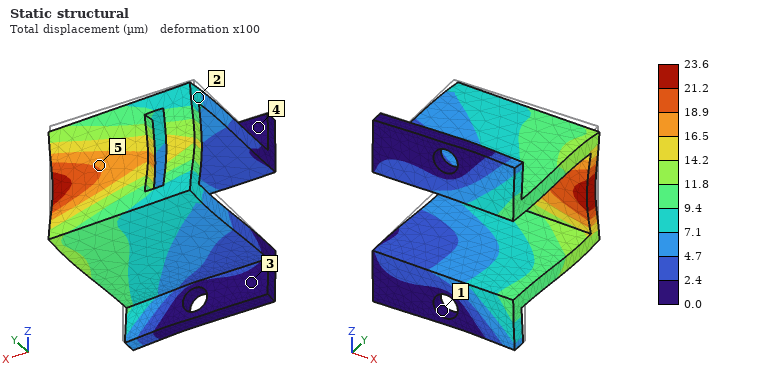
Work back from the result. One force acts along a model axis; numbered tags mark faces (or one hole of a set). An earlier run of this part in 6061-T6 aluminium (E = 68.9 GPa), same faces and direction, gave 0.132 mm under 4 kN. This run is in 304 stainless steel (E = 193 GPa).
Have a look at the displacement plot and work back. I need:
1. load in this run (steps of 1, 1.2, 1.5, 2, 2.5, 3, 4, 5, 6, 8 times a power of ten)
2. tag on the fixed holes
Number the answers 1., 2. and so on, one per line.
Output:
1. 2 kN
2. 1
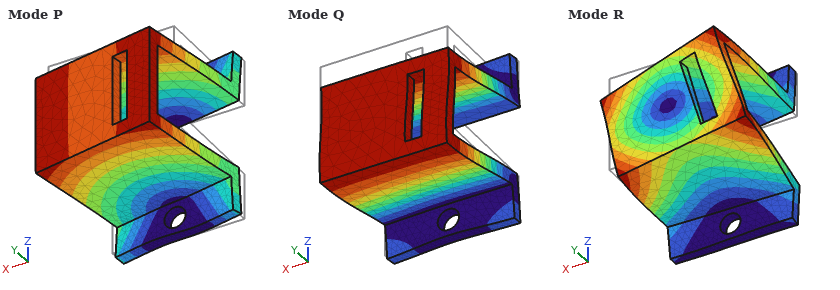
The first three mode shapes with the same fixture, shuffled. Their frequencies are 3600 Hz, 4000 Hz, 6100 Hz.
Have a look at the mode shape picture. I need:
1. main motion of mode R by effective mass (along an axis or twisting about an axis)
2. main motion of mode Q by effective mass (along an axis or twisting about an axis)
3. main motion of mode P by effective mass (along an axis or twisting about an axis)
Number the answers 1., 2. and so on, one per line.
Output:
1. twisting about Y
2. along Z
3. along X
